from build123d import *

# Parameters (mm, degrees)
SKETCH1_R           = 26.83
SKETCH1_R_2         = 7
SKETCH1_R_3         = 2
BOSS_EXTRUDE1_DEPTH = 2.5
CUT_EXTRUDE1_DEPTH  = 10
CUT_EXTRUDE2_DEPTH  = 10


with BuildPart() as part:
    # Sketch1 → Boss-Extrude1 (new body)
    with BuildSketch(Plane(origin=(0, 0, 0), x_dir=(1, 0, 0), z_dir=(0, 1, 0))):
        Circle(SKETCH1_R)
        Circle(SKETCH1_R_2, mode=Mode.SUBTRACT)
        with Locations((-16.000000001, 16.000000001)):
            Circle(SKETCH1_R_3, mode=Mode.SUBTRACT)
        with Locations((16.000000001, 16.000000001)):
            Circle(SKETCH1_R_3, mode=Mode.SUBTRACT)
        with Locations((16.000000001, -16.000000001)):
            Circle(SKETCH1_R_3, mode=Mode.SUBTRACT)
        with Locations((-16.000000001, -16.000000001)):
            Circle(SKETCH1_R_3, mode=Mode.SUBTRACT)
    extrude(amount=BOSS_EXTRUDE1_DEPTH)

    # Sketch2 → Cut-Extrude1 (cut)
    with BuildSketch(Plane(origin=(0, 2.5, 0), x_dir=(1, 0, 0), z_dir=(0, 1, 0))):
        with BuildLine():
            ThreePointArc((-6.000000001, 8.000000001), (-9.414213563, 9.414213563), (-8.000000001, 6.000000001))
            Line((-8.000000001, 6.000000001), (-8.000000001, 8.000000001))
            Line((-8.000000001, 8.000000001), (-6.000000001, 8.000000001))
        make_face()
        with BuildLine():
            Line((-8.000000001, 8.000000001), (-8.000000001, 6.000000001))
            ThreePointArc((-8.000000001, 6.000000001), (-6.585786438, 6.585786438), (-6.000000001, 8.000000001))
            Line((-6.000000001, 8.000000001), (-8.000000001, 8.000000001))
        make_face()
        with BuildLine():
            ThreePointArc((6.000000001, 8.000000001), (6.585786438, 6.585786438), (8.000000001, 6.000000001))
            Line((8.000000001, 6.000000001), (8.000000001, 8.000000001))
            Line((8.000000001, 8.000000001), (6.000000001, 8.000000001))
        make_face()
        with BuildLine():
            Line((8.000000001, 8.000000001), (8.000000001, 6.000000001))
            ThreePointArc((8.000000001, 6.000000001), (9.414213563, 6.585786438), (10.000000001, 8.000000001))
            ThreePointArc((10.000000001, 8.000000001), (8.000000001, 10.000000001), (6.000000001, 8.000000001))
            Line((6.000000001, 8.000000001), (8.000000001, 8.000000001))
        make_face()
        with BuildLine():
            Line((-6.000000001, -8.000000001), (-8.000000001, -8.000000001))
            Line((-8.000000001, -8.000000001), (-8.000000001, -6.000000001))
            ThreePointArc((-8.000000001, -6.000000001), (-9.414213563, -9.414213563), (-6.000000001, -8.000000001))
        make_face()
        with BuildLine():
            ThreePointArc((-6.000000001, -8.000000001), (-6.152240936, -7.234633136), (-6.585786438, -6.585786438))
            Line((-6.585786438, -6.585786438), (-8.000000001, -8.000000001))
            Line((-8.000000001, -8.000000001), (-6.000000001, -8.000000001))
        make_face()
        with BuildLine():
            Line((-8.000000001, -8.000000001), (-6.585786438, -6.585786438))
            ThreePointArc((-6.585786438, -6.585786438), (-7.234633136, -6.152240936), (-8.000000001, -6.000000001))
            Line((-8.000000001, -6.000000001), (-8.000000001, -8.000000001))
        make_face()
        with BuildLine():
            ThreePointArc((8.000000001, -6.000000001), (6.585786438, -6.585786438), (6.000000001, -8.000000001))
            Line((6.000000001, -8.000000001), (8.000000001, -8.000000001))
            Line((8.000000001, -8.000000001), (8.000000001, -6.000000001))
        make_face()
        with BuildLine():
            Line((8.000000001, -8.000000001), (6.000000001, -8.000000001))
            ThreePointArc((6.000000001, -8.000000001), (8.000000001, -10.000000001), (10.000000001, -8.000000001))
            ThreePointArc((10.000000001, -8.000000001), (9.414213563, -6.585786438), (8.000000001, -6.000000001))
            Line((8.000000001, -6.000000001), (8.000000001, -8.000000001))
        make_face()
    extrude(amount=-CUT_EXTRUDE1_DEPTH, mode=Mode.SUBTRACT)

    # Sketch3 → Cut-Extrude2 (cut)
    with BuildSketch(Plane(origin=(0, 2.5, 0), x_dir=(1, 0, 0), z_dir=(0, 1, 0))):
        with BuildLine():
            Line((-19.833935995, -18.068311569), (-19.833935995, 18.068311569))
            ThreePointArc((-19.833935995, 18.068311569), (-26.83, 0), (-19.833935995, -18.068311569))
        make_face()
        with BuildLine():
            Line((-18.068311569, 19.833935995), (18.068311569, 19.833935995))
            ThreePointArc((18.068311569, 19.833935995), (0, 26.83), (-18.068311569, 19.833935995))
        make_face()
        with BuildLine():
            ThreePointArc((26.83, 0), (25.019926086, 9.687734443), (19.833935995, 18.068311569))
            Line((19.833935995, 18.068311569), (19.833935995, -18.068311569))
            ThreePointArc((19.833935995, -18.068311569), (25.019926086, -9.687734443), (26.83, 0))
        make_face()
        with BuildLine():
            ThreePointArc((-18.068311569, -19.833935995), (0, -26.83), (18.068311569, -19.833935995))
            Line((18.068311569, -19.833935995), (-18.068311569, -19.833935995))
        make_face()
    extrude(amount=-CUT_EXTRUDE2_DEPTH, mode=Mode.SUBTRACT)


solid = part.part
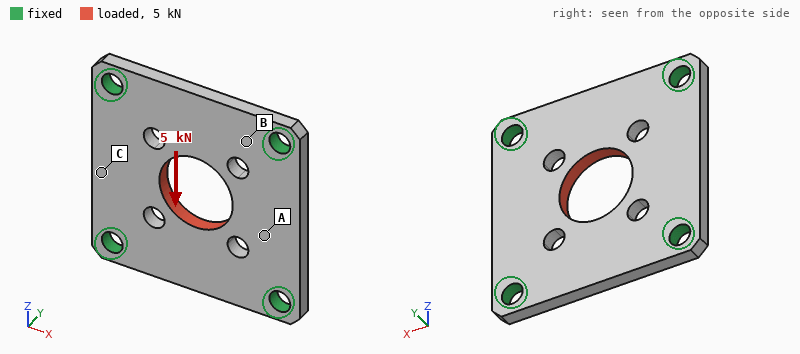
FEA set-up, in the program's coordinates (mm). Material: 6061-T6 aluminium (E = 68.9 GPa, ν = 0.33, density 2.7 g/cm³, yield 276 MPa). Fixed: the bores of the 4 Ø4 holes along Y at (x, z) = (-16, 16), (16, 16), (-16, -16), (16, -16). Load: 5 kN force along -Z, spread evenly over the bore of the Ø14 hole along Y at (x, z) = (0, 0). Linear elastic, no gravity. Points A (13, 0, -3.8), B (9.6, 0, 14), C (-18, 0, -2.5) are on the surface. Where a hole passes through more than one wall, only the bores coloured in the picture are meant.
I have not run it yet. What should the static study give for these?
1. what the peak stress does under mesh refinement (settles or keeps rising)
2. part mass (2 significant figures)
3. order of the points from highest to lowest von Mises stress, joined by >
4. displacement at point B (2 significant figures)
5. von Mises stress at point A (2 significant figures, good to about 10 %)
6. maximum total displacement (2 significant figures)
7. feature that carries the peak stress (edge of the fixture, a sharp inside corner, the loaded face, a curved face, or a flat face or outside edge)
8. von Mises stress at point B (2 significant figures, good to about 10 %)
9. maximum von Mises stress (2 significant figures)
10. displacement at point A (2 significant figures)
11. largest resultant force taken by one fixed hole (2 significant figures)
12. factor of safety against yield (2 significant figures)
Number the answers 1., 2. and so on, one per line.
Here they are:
1. settles
2. 8.9 g
3. B > A > C
4. 8.2 µm
5. 31 MPa
6. 20 µm
7. a curved face
8. 55 MPa
9. 150 MPa
10. 7.0 µm
11. 1.4 kN
12. 1.8
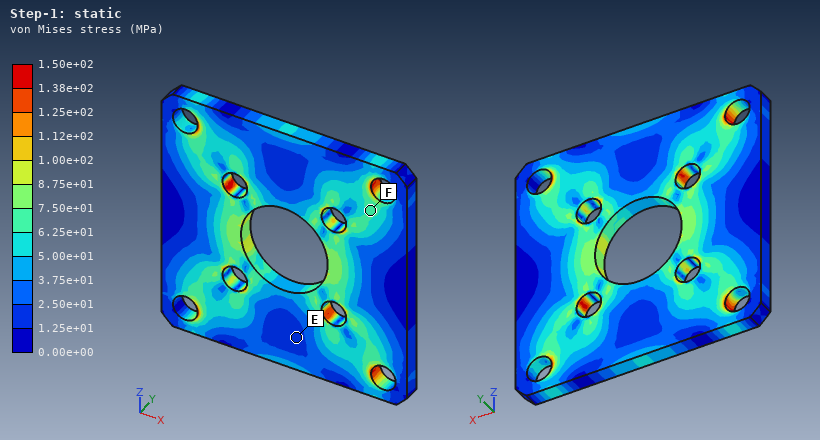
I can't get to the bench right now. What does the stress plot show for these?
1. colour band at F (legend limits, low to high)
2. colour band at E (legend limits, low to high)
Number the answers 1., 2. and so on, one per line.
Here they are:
1. 6.25e+01 to 7.50e+01 MPa
2. 1.25e+01 to 2.50e+01 MPa
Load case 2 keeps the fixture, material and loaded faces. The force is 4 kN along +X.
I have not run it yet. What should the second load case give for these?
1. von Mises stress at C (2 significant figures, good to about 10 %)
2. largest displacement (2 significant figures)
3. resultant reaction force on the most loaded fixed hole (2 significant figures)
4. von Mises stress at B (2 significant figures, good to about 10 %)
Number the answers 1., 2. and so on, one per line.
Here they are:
1. 23 MPa
2. 16 µm
3. 1.1 kN
4. 48 MPa
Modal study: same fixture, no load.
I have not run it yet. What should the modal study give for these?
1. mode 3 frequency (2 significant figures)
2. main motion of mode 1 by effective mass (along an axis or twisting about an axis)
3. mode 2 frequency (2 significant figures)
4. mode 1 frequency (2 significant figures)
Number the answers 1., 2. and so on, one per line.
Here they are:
1. 15 kHz
2. along Y
3. 15 kHz
4. 11 kHz
